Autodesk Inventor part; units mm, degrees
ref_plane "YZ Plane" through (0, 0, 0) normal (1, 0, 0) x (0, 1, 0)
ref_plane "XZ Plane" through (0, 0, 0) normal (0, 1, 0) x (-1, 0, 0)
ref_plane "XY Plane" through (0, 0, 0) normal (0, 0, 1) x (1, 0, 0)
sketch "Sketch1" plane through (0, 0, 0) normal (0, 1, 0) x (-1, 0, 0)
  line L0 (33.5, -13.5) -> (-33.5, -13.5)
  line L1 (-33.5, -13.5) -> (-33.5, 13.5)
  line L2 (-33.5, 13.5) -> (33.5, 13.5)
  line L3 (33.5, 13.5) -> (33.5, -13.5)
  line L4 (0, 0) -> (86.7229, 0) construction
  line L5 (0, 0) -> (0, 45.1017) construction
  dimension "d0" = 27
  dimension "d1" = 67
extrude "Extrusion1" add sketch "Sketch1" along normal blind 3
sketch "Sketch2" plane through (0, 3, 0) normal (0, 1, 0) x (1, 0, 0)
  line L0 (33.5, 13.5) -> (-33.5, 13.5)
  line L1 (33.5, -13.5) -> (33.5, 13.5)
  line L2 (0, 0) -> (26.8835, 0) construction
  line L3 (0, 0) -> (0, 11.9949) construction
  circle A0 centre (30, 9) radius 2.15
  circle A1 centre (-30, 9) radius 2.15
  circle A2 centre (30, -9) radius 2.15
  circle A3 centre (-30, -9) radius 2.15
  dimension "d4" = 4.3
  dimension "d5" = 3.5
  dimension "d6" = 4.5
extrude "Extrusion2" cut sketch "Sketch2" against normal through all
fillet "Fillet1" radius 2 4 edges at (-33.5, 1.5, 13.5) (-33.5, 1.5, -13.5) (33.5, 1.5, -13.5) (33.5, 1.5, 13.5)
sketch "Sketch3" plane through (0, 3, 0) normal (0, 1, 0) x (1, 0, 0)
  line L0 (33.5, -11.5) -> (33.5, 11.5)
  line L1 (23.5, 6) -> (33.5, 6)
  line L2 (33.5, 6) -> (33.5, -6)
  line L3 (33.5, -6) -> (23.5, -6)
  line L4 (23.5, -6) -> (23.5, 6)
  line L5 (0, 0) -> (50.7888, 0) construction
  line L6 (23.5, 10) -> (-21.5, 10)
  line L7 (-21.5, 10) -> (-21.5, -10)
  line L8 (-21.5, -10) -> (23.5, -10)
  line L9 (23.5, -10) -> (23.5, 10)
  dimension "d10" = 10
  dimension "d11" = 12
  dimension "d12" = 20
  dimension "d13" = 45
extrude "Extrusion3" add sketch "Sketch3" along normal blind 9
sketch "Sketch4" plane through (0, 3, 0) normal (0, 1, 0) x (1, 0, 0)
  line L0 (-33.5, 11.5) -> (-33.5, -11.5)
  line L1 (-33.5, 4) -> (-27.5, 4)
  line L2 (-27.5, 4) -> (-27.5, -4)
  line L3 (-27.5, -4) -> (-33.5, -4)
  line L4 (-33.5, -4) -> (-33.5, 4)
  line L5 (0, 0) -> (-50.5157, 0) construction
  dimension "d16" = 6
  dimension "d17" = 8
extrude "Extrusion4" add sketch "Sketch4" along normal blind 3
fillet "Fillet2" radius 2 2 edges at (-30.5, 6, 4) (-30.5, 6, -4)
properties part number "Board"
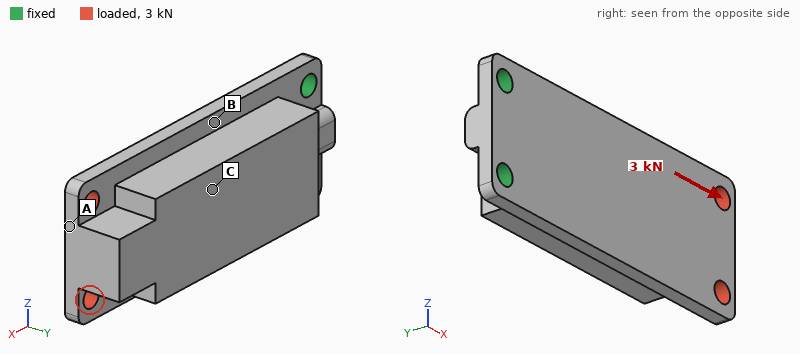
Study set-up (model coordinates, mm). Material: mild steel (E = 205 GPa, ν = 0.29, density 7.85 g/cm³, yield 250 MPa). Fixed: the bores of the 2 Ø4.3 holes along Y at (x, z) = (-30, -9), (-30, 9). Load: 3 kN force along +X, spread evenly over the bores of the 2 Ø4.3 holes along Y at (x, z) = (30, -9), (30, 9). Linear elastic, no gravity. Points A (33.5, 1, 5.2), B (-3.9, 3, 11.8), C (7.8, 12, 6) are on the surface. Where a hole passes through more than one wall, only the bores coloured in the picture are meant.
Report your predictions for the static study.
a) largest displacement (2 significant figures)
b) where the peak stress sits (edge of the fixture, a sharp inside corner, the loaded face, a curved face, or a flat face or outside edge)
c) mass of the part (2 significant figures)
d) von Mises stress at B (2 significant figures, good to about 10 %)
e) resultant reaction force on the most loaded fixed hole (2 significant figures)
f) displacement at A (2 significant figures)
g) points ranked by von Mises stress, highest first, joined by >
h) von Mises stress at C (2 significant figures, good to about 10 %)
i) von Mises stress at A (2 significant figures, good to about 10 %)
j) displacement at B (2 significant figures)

34 µm
the loaded face
110 g
22 MPa
1.5 kN
33 µm
A > B > C
12 MPa
59 MPa
5.4 µm
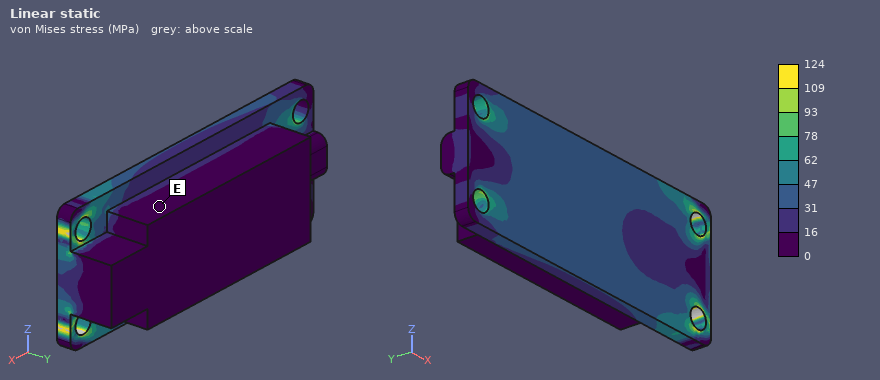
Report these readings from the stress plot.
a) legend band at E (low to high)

0 to 16 MPa
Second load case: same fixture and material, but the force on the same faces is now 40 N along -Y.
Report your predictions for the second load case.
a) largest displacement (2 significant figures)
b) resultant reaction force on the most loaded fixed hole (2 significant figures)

96 µm
26 N
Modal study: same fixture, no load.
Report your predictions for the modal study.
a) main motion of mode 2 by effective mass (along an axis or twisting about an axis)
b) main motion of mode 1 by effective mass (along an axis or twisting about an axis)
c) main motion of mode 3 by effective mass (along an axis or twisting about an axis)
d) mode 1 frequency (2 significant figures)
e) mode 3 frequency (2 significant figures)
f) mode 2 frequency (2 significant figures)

along Z
along Y
twisting about X
540 Hz
5600 Hz
3400 Hz
